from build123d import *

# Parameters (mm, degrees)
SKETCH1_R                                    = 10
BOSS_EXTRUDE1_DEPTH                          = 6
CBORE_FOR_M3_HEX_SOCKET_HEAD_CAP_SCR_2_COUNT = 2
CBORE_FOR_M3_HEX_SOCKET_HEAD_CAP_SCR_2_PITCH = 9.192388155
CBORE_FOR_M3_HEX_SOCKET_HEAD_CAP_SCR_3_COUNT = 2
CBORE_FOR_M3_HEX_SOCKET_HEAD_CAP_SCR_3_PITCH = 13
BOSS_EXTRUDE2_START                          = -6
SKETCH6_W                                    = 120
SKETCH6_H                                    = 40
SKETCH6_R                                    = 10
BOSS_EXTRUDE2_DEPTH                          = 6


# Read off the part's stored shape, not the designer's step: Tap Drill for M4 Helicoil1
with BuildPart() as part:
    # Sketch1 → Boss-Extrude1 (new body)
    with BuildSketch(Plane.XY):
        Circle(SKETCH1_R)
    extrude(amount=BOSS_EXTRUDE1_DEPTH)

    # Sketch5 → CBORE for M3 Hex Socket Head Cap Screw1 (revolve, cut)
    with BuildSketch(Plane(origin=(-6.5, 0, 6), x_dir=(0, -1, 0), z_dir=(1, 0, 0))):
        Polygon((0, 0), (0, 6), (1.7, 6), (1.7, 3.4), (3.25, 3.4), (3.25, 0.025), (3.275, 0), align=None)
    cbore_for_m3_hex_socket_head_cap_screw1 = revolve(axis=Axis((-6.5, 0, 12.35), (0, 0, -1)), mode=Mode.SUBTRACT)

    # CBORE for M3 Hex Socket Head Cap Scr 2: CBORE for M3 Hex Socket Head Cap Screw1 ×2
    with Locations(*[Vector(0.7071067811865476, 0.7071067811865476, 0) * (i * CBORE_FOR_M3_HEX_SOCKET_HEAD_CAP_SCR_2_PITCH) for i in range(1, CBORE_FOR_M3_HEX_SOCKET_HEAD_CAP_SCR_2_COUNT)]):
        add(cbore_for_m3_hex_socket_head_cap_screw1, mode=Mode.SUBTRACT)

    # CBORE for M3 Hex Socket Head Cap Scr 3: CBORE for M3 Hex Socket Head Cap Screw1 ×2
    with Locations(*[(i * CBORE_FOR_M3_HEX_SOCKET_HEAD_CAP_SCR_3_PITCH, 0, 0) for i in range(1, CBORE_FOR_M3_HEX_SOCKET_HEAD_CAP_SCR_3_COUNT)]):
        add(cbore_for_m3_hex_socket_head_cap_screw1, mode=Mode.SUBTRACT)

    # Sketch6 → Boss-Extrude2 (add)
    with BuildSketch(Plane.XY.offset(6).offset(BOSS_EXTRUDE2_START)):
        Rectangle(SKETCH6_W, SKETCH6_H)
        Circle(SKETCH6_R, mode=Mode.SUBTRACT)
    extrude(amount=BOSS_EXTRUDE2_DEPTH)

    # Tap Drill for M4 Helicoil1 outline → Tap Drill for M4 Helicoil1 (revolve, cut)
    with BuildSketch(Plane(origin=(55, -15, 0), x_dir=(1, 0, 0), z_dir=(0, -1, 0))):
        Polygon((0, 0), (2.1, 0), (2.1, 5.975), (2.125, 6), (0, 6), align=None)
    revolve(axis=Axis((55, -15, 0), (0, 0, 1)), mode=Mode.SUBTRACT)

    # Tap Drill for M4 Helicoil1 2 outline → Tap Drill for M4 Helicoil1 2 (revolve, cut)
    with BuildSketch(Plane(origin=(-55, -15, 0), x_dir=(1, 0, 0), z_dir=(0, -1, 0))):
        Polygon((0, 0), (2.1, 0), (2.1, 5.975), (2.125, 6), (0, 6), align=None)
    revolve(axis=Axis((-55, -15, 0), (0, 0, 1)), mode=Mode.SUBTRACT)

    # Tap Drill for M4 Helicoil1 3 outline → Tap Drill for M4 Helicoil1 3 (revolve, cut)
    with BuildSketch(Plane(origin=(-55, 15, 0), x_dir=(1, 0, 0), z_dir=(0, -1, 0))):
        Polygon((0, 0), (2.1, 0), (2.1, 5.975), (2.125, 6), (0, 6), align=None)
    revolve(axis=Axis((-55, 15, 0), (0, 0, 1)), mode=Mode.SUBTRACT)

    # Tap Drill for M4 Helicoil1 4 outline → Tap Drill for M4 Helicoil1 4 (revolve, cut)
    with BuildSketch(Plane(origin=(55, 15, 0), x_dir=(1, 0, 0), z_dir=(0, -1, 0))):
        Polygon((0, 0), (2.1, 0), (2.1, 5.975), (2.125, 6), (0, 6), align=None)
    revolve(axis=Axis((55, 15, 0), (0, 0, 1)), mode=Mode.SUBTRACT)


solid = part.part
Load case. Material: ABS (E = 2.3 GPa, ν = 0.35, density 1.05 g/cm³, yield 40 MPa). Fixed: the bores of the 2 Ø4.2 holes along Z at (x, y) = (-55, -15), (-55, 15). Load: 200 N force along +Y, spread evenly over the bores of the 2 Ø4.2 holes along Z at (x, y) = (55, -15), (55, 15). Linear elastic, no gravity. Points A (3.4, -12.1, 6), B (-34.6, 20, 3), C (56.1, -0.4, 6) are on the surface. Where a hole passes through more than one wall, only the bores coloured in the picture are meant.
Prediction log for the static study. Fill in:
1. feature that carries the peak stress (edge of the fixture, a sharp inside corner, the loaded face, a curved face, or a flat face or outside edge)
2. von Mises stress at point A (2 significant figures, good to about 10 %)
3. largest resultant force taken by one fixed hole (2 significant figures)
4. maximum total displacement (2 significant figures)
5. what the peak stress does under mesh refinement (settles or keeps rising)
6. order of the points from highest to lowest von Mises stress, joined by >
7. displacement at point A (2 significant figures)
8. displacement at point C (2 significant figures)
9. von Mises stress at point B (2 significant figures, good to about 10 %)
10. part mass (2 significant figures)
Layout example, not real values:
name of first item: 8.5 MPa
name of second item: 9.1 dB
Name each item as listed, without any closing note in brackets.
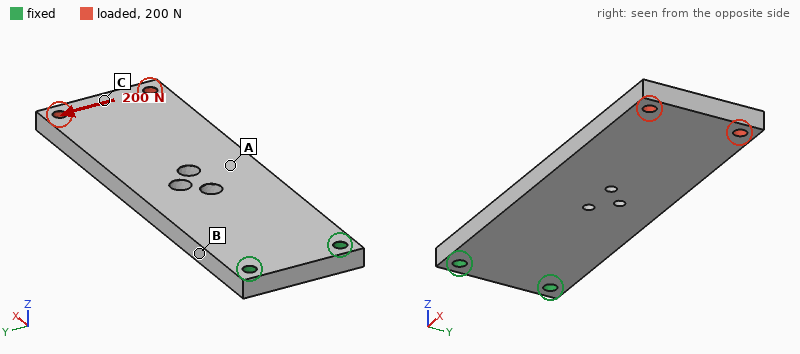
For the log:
feature that carries the peak stress: edge of the fixture
von Mises stress at point A: 4.2 MPa
largest resultant force taken by one fixed hole: 710 N
maximum total displacement: 1.5 mm
what the peak stress does under mesh refinement: keeps rising
order of the points from highest to lowest von Mises stress, joined by >: B > A > C
displacement at point A: 0.52 mm
displacement at point C: 1.4 mm
von Mises stress at point B: 11 MPa
part mass: 29 g
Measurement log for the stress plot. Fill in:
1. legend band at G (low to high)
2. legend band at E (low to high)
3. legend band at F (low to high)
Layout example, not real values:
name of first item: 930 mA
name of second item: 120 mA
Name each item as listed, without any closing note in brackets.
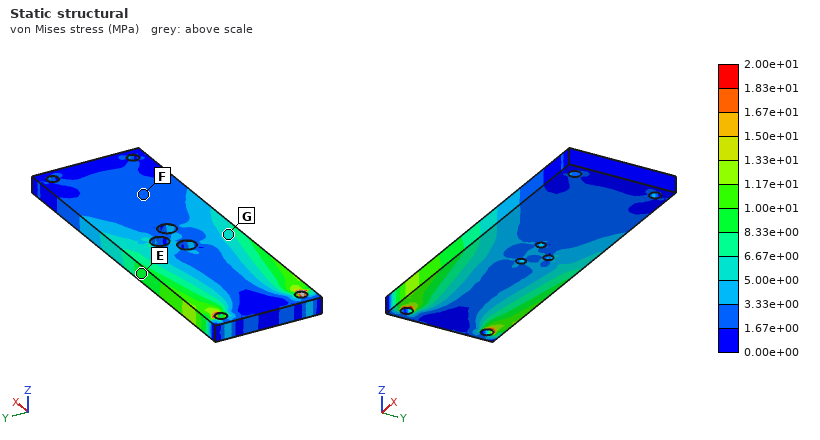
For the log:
legend band at G: 5.00e+00 to 6.67e+00 MPa
legend band at E: 8.33e+00 to 1.00e+01 MPa
legend band at F: 1.67e+00 to 3.33e+00 MPa
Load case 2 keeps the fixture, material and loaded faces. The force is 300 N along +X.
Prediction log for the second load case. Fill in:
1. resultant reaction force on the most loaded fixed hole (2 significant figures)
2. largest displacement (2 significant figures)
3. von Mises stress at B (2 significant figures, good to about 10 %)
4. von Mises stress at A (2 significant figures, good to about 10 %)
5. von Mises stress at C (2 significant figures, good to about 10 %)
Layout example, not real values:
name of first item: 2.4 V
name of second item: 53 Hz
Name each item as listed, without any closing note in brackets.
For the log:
resultant reaction force on the most loaded fixed hole: 150 N
largest displacement: 85 µm
von Mises stress at B: 1.4 MPa
von Mises stress at A: 1.5 MPa
von Mises stress at C: 0.67 MPa
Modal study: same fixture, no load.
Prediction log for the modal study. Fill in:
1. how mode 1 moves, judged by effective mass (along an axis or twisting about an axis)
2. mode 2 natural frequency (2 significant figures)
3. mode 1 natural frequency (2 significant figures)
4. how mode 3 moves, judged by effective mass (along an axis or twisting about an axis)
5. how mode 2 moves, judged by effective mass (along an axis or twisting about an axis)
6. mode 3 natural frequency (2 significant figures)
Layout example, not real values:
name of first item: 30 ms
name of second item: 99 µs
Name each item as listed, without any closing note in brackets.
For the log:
how mode 1 moves, judged by effective mass: along Z
mode 2 natural frequency: 600 Hz
mode 1 natural frequency: 110 Hz
how mode 3 moves, judged by effective mass: along Z
how mode 2 moves, judged by effective mass: twisting about X
mode 3 natural frequency: 650 Hz
